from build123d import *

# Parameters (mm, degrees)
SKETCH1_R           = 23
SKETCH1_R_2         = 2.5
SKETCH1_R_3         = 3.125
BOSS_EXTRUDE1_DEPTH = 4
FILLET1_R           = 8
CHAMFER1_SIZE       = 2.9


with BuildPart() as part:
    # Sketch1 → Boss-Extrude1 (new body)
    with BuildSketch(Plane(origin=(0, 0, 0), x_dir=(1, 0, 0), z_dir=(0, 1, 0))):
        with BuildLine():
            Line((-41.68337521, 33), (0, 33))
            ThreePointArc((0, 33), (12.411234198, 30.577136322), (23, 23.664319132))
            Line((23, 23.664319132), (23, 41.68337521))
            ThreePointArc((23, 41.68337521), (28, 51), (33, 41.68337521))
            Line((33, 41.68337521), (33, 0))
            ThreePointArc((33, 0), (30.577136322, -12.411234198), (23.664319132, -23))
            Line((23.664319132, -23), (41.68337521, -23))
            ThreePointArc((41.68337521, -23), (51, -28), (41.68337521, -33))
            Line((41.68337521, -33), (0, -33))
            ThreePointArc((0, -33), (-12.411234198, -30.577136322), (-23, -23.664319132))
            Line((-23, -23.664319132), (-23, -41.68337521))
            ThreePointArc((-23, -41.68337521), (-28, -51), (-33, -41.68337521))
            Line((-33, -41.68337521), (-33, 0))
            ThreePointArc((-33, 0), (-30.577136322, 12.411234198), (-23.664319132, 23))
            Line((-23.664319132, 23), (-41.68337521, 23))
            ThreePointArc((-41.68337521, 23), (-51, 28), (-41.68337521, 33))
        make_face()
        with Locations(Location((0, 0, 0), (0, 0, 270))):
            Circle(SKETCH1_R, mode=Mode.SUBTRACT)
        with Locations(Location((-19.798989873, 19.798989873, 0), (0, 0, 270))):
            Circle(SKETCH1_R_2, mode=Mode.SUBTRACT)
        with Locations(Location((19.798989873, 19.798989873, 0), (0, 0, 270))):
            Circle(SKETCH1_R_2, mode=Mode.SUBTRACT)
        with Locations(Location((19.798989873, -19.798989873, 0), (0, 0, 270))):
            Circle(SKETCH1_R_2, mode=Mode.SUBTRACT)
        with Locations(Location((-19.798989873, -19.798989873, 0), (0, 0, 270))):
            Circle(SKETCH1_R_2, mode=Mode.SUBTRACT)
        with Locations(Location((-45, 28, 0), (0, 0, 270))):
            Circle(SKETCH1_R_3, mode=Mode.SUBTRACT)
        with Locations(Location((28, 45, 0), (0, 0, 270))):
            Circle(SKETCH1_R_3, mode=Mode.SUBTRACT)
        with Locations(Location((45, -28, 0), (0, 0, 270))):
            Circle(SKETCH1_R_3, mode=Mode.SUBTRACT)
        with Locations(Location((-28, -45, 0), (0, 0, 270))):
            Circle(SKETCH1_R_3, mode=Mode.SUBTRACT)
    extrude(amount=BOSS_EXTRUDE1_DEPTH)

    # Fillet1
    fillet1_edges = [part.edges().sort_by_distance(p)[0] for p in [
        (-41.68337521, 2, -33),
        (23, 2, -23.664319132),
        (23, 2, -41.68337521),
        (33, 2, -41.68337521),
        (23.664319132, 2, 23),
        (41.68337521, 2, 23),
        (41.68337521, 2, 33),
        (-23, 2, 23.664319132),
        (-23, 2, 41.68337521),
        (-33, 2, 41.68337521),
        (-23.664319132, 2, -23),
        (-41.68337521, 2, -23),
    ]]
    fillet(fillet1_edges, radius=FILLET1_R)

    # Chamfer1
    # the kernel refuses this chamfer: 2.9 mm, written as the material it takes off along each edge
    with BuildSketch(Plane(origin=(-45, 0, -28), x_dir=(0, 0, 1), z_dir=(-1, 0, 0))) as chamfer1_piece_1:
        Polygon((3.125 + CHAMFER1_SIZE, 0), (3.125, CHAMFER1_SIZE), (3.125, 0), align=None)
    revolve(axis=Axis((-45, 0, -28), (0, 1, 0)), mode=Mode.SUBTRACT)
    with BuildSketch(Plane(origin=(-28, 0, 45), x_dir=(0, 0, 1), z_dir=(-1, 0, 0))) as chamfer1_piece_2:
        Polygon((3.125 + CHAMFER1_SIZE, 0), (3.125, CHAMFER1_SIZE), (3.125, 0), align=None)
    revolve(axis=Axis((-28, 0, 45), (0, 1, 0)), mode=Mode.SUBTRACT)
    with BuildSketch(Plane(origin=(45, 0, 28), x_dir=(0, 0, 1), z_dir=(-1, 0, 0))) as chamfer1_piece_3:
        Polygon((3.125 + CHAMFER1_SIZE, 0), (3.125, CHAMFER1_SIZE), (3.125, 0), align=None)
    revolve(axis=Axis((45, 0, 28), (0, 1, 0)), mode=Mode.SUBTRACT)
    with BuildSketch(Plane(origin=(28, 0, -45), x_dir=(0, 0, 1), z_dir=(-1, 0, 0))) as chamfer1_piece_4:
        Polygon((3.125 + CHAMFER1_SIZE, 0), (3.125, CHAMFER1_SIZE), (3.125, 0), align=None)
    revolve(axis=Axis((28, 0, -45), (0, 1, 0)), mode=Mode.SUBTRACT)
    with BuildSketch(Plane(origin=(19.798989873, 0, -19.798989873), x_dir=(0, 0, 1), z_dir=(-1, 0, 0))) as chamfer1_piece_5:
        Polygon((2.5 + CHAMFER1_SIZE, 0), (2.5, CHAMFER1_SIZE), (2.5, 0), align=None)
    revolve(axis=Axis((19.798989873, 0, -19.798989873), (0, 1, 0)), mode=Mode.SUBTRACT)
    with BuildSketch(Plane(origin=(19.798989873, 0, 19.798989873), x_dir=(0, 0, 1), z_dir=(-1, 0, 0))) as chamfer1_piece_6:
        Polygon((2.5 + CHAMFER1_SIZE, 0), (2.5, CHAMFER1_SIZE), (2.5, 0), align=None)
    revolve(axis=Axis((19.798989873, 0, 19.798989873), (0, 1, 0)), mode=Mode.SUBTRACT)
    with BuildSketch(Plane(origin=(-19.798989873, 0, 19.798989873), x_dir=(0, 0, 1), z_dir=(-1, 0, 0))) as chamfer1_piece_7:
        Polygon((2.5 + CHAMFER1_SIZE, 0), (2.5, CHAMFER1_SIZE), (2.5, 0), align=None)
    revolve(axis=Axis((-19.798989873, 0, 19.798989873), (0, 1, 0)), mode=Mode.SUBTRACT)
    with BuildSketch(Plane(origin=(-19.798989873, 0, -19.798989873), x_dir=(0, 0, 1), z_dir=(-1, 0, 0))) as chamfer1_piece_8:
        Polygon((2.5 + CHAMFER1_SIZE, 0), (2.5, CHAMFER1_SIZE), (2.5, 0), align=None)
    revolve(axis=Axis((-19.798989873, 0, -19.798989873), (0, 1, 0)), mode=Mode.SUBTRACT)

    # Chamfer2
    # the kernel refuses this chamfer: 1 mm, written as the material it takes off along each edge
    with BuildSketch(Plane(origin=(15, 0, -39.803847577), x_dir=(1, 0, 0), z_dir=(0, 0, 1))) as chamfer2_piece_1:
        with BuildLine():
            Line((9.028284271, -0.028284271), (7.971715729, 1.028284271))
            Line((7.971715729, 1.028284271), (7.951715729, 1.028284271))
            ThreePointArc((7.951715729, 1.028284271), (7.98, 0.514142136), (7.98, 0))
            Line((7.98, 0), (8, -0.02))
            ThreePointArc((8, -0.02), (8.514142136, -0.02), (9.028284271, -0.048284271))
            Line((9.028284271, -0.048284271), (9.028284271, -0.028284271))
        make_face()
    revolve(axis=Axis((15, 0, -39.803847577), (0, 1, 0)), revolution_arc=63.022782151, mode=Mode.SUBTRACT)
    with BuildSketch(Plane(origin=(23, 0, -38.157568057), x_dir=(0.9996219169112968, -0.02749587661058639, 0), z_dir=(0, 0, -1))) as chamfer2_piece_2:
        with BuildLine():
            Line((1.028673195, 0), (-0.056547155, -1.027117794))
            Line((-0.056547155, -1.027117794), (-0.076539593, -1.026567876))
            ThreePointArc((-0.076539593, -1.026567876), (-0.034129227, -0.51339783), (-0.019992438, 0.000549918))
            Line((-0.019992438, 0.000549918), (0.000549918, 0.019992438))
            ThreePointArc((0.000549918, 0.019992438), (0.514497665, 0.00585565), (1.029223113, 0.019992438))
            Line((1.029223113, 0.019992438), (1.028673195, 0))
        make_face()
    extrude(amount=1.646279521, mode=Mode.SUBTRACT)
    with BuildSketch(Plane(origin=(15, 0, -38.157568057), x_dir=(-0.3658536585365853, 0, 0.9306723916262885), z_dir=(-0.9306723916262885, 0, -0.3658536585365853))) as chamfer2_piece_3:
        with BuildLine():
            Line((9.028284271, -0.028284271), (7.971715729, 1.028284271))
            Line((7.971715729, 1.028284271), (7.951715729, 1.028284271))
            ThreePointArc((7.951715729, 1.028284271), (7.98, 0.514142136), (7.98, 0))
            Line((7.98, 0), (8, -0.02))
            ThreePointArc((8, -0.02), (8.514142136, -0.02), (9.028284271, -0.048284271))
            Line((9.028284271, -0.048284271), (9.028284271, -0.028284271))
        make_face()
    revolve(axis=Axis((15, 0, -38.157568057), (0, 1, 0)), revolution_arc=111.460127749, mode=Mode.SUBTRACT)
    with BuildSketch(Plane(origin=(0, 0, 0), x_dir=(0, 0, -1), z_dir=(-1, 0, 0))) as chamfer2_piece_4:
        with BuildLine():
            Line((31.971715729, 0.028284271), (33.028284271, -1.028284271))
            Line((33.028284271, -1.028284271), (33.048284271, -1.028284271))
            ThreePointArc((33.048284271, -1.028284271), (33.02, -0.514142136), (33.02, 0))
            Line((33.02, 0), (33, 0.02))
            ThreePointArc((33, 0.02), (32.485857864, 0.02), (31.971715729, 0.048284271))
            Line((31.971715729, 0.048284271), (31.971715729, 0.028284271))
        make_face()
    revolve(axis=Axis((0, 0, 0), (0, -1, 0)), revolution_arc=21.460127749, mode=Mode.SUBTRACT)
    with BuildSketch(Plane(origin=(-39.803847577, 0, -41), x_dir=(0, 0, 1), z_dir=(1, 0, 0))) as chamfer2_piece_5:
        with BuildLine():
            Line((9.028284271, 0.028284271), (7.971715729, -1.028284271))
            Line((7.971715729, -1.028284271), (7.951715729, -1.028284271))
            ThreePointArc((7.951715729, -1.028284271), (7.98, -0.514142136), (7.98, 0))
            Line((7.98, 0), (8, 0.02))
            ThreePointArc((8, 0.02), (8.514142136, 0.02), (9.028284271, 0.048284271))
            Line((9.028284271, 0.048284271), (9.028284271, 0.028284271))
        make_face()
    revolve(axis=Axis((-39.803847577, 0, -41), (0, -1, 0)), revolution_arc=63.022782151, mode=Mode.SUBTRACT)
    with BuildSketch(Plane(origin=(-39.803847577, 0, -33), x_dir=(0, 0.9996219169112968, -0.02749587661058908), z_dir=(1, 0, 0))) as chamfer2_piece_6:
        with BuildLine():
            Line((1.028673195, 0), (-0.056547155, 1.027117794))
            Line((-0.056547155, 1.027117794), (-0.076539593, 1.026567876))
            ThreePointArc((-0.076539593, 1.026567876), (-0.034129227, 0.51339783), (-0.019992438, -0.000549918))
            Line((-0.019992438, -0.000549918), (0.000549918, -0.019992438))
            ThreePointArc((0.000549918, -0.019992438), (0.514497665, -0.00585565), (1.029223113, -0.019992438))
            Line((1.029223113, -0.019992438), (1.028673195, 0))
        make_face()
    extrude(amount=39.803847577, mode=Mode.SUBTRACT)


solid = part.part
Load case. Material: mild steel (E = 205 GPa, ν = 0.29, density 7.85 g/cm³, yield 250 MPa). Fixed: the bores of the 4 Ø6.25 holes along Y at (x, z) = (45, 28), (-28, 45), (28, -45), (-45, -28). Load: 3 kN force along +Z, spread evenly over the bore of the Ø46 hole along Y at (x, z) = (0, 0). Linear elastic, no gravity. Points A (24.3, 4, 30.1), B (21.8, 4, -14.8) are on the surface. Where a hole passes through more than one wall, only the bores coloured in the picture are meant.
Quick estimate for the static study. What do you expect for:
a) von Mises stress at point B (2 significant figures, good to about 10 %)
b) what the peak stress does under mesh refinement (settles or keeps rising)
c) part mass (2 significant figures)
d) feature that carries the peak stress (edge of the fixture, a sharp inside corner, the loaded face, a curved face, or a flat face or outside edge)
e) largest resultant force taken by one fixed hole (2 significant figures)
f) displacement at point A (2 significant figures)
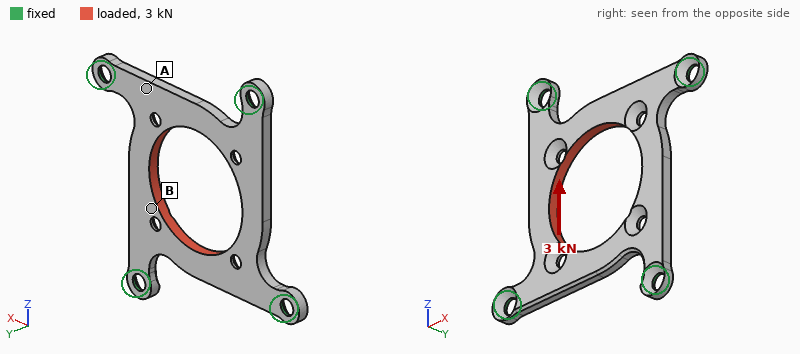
29 MPa
keeps rising
91 g
edge of the fixture
1.2 kN
7.5 µm
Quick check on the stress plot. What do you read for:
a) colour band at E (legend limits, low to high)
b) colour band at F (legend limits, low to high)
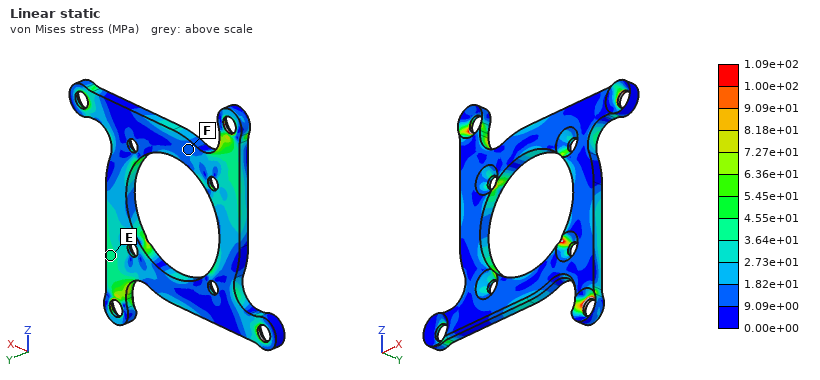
3.64e+01 to 4.55e+01 MPa
9.09e+00 to 1.82e+01 MPa
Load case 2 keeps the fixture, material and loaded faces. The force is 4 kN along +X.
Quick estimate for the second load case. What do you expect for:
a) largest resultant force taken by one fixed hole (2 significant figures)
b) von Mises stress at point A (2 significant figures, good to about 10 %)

1.6 kN
51 MPa
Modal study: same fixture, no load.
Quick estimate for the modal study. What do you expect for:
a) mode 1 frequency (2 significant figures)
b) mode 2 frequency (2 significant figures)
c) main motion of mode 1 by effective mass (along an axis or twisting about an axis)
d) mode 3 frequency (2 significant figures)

2000 Hz
3100 Hz
along Y
3100 Hz
